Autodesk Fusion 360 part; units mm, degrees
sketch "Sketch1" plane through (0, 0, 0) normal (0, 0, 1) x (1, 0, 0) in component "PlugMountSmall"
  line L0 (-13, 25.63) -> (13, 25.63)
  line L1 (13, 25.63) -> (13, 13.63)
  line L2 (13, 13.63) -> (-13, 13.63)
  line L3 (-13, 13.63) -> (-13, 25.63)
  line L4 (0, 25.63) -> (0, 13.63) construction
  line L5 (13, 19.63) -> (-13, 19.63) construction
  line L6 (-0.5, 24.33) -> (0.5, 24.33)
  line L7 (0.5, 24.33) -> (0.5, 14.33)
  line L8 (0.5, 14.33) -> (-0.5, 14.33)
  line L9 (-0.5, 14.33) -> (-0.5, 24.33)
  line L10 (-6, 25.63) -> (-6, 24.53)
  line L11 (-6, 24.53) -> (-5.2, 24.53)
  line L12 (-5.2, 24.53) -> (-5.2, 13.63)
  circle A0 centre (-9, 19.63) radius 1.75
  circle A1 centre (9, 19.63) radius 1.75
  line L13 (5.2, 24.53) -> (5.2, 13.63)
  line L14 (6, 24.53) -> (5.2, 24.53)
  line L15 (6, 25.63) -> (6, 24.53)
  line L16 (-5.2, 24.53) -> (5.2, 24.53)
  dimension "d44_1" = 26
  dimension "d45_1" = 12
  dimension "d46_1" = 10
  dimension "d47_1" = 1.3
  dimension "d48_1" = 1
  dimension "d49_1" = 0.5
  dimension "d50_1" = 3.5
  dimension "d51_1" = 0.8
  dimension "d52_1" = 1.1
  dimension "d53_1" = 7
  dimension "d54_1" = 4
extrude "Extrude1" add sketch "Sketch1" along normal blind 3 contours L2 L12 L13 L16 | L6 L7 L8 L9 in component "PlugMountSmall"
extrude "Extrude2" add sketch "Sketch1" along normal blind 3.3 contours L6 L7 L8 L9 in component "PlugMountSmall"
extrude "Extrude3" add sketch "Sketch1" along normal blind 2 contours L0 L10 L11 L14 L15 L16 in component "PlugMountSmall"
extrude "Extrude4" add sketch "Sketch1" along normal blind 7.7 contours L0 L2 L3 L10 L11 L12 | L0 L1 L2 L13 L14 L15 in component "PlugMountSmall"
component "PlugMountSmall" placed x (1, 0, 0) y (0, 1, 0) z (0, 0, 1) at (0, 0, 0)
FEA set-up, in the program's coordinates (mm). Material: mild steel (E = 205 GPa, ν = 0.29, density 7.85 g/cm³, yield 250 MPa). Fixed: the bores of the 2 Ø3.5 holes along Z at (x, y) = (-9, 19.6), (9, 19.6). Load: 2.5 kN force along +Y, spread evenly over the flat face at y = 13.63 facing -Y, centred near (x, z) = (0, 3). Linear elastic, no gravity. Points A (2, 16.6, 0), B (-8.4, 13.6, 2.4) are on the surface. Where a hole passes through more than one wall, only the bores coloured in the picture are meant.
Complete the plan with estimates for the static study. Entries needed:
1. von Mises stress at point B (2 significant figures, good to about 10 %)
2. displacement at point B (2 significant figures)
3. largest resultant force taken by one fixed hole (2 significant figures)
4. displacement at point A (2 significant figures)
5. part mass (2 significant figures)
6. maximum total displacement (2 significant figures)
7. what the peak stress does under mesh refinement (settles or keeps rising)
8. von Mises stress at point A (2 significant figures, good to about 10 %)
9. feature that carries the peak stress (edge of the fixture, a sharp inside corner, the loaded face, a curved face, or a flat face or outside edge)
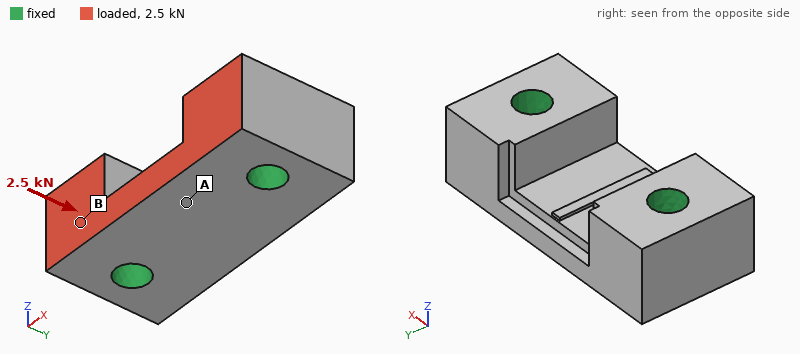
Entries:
22 MPa
0.49 µm
1.3 kN
0.94 µm
13 g
1.2 µm
keeps rising
13 MPa
edge of the fixture
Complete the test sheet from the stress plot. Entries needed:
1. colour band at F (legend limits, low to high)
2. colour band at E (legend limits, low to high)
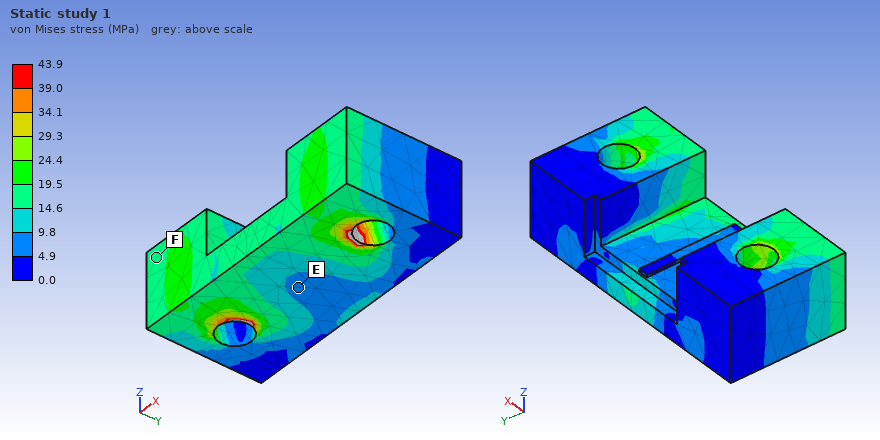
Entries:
14.6 to 19.5 MPa
4.9 to 9.8 MPa
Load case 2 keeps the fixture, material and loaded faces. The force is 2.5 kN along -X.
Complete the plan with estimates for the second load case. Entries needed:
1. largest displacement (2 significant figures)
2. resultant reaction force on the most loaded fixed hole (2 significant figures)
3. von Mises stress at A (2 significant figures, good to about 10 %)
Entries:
2.9 µm
1.3 kN
33 MPa
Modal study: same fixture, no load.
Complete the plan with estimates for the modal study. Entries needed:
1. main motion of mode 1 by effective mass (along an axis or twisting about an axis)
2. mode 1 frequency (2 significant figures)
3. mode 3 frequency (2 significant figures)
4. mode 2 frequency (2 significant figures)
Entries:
along Z
65 kHz
79 kHz
70 kHz
